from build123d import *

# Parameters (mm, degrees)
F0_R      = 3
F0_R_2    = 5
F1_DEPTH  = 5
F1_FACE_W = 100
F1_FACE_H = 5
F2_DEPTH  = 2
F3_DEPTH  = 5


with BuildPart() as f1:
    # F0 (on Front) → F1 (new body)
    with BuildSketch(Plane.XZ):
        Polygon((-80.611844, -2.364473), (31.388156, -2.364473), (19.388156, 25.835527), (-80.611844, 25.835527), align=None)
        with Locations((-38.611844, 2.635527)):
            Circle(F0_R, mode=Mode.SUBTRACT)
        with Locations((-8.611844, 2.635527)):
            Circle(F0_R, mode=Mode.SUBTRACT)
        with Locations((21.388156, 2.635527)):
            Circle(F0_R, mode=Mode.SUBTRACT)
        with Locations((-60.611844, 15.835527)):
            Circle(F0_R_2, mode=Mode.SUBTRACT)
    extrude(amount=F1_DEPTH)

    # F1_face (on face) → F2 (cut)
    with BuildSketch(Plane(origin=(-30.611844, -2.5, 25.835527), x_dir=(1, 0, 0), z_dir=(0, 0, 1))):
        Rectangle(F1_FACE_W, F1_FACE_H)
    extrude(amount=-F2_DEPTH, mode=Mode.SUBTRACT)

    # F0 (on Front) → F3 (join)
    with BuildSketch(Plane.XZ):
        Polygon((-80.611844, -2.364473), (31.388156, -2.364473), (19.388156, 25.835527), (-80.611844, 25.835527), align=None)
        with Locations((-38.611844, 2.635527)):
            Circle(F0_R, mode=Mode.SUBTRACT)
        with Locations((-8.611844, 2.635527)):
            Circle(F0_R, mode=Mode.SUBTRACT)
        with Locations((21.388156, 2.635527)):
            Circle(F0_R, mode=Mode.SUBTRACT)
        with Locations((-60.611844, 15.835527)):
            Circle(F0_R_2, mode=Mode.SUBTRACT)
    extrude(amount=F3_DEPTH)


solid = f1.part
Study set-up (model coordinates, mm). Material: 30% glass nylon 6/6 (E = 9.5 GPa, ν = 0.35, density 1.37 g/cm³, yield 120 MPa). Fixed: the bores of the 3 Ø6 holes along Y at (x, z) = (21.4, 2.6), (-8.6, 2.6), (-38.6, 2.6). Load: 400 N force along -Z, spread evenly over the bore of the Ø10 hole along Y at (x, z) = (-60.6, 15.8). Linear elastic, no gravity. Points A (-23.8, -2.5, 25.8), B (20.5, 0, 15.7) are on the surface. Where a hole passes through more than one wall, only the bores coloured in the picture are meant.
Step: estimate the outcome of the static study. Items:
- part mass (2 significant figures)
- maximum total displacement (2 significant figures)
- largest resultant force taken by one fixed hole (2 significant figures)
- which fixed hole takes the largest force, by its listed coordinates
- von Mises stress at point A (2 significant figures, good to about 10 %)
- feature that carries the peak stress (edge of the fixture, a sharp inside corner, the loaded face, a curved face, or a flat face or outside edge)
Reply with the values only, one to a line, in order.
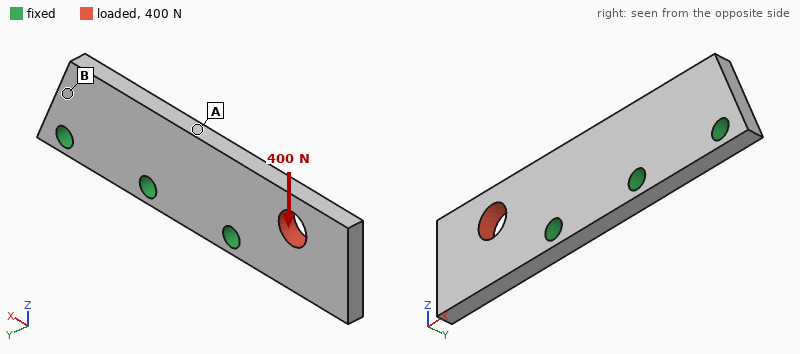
19 g
0.11 mm
610 N
(-38.6, 2.6)
5.7 MPa
edge of the fixture
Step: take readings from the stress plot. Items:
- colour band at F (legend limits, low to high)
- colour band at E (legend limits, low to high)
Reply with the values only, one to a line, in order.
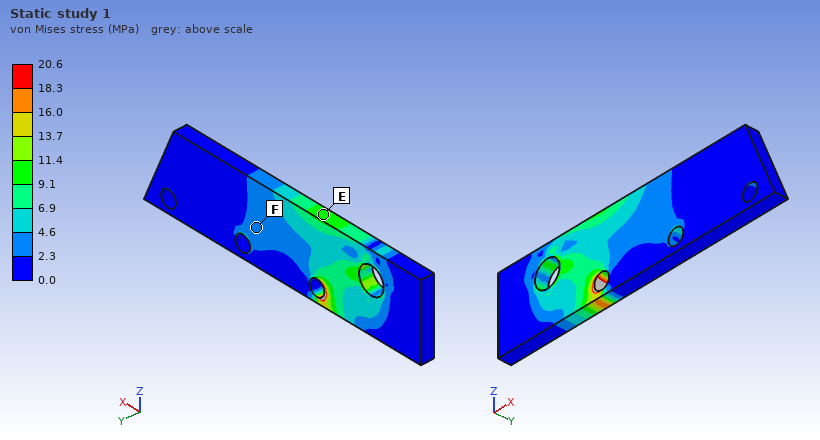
2.3 to 4.6 MPa
9.1 to 11.4 MPa
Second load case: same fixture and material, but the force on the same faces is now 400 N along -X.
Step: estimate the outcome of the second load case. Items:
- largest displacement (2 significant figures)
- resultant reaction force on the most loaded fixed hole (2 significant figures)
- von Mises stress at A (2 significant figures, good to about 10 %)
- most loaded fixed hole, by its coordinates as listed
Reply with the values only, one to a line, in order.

49 µm
240 N
3.3 MPa
(-38.6, 2.6)
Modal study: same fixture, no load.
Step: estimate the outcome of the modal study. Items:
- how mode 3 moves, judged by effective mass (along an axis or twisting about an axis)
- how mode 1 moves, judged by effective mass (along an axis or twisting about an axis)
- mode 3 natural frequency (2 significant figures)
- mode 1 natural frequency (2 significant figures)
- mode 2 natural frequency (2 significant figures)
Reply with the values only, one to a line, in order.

along Z
along Y
4000 Hz
1100 Hz
2800 Hz
